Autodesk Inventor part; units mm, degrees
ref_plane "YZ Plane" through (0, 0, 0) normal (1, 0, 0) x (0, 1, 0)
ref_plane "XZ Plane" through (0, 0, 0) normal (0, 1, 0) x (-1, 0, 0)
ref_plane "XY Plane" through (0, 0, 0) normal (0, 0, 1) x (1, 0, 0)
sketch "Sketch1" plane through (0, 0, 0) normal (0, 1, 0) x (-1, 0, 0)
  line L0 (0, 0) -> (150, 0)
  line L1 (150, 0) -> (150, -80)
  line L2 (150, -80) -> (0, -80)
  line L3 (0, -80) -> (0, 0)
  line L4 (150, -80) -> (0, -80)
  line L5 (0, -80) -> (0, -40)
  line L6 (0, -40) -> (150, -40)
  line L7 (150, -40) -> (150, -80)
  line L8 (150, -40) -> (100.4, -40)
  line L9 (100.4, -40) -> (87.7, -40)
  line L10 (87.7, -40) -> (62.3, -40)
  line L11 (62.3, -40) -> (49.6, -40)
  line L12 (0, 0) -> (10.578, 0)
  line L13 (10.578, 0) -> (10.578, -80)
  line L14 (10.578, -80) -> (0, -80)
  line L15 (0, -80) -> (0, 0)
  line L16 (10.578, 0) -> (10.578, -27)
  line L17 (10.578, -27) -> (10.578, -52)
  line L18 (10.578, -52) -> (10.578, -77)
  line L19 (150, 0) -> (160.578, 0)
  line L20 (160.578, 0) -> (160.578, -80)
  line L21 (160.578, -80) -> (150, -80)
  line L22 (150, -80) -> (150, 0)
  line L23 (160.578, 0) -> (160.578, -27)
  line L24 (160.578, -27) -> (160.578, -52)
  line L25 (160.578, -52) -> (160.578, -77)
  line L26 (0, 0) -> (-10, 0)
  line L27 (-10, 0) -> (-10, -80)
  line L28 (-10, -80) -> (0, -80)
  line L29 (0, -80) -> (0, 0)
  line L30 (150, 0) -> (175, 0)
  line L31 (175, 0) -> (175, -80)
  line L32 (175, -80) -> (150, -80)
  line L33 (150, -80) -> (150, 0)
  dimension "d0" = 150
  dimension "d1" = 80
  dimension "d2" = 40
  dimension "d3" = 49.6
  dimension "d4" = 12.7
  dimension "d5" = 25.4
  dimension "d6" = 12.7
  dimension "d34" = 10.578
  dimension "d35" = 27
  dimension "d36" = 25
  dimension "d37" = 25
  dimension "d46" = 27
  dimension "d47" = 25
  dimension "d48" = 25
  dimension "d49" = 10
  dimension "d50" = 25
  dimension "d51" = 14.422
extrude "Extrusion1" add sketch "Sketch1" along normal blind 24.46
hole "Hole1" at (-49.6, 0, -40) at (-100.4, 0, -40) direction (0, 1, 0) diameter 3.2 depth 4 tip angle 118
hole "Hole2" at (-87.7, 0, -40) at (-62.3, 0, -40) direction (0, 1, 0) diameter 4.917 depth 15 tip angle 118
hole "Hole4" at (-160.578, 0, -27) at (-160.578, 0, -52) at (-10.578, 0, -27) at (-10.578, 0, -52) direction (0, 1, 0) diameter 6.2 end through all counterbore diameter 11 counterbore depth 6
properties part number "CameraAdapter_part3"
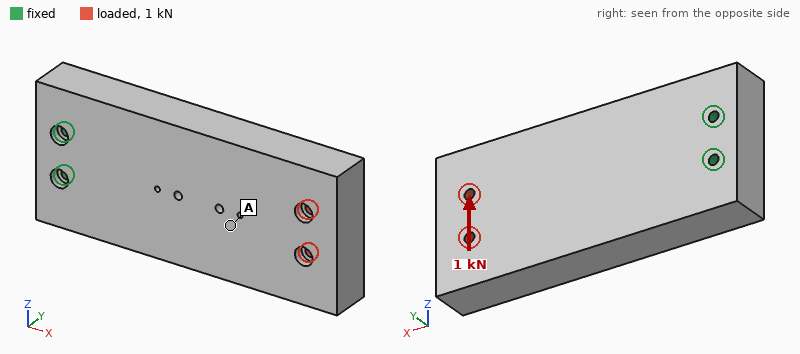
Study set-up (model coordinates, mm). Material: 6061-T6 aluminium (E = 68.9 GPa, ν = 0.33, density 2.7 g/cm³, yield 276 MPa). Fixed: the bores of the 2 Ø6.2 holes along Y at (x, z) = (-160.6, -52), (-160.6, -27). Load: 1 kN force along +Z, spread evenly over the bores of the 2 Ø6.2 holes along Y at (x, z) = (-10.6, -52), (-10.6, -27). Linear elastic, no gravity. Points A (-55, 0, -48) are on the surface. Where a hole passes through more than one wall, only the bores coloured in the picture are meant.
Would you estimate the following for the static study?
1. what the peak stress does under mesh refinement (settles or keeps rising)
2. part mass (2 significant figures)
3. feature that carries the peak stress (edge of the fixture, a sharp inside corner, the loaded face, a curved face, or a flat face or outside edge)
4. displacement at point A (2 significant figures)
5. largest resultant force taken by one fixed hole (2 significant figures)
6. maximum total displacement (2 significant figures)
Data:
keeps rising
960 g
edge of the fixture
30 µm
5.1 kN
56 µm
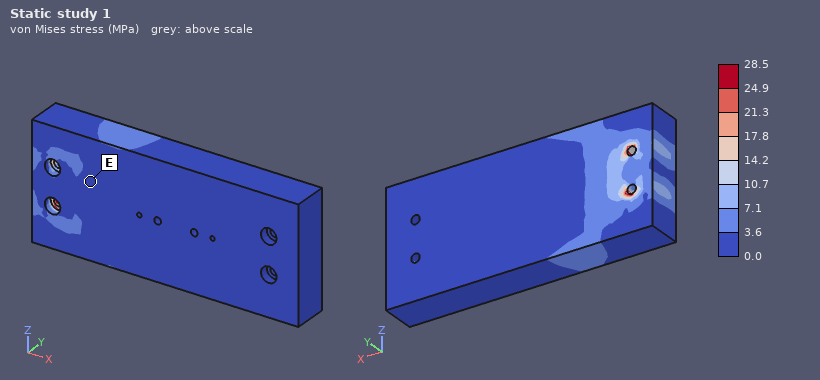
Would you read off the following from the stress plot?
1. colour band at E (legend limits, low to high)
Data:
0.0 to 3.6 MPa
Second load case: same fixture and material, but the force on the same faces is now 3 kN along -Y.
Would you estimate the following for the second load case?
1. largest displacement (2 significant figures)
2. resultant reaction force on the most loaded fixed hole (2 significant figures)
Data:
0.84 mm
1.7 kN
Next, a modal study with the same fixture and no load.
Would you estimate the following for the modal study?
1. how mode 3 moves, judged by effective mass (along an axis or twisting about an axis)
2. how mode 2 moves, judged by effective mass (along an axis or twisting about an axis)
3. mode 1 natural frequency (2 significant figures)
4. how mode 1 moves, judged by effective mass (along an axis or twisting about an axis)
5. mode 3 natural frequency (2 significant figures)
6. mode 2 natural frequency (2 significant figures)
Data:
twisting about X
along Z
570 Hz
along Y
2300 Hz
1200 Hz
